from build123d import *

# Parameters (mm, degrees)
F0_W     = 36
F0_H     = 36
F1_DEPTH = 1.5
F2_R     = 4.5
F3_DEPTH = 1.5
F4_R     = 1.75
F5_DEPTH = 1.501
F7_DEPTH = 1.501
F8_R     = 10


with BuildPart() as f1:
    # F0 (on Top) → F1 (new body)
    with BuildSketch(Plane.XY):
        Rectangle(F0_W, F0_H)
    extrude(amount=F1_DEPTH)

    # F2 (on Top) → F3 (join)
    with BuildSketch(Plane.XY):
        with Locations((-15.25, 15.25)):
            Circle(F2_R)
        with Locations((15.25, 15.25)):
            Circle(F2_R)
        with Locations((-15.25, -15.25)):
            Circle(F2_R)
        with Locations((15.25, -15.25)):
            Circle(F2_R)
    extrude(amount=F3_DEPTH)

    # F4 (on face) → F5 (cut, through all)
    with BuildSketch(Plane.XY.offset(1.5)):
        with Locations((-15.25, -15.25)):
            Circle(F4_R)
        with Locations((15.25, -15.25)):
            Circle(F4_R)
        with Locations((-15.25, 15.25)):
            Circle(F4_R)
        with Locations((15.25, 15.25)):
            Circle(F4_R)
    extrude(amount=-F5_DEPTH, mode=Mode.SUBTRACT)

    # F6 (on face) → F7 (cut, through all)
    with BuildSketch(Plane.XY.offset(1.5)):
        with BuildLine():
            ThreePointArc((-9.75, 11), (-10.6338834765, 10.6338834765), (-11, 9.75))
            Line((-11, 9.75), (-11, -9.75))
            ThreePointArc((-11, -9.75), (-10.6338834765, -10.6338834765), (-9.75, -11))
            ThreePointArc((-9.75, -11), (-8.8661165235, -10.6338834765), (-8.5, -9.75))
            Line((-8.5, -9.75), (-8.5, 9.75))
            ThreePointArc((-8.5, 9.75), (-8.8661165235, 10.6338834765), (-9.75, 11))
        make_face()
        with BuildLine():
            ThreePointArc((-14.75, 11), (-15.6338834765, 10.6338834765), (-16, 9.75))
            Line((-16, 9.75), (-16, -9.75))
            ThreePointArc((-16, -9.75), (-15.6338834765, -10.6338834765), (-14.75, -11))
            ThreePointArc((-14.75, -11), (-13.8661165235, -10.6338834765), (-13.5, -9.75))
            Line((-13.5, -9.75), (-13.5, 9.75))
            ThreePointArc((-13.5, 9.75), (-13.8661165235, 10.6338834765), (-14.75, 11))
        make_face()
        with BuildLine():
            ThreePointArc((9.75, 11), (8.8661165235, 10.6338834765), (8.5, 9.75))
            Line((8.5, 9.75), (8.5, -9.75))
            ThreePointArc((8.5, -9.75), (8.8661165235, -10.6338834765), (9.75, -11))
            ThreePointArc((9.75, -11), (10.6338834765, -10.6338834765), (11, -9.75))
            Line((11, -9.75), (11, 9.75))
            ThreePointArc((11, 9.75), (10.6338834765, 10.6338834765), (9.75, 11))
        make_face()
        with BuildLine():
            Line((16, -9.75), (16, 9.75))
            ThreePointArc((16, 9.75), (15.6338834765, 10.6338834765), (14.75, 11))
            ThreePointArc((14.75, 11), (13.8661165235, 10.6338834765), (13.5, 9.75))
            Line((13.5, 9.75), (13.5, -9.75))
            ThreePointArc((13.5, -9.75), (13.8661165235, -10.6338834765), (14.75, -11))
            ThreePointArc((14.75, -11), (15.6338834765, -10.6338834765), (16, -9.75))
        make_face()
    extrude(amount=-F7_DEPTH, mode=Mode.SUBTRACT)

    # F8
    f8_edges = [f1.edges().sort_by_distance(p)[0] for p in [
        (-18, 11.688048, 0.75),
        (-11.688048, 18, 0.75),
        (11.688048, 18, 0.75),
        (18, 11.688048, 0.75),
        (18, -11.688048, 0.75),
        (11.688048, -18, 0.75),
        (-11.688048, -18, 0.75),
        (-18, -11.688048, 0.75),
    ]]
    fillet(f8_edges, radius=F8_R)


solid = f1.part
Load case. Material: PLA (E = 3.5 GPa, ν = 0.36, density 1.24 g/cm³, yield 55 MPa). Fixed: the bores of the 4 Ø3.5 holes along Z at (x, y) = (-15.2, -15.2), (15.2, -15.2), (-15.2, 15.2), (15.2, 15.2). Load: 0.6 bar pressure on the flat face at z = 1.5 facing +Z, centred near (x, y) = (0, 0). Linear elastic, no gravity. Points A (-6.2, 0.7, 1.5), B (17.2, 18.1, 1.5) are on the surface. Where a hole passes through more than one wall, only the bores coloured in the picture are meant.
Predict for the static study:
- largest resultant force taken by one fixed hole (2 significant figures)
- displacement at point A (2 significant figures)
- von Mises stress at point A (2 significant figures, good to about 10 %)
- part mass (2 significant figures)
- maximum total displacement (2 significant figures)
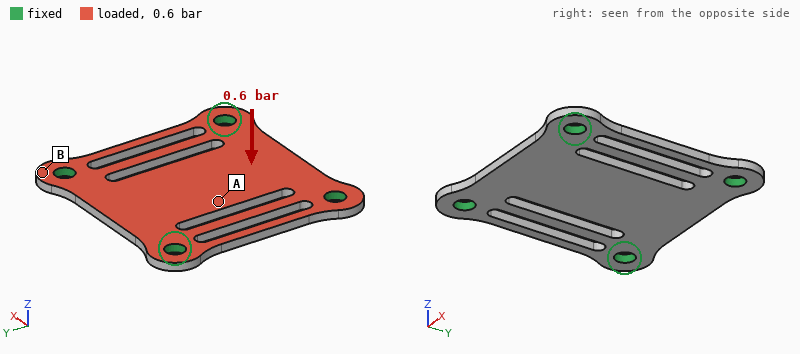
17 N
0.32 mm
8.3 MPa
2.1 g
0.33 mm
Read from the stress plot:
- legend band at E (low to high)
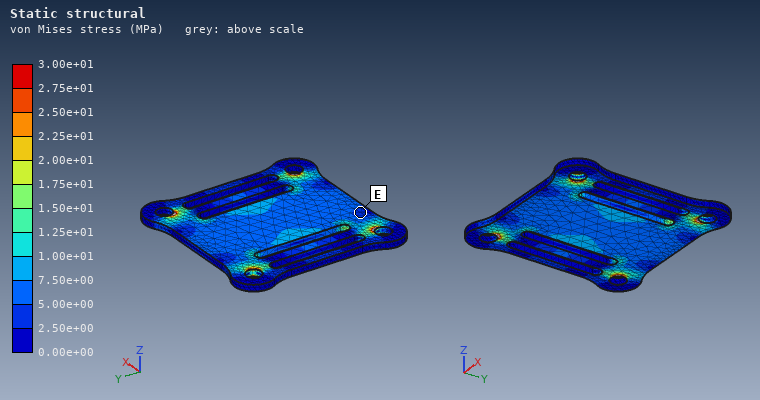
2.50e+00 to 5.00e+00 MPa
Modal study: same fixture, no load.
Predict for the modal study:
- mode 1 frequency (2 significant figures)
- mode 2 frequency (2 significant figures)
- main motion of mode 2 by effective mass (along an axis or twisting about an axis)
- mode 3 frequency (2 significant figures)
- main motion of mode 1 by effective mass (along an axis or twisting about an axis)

1800 Hz
3400 Hz
twisting about X
3600 Hz
along Z
